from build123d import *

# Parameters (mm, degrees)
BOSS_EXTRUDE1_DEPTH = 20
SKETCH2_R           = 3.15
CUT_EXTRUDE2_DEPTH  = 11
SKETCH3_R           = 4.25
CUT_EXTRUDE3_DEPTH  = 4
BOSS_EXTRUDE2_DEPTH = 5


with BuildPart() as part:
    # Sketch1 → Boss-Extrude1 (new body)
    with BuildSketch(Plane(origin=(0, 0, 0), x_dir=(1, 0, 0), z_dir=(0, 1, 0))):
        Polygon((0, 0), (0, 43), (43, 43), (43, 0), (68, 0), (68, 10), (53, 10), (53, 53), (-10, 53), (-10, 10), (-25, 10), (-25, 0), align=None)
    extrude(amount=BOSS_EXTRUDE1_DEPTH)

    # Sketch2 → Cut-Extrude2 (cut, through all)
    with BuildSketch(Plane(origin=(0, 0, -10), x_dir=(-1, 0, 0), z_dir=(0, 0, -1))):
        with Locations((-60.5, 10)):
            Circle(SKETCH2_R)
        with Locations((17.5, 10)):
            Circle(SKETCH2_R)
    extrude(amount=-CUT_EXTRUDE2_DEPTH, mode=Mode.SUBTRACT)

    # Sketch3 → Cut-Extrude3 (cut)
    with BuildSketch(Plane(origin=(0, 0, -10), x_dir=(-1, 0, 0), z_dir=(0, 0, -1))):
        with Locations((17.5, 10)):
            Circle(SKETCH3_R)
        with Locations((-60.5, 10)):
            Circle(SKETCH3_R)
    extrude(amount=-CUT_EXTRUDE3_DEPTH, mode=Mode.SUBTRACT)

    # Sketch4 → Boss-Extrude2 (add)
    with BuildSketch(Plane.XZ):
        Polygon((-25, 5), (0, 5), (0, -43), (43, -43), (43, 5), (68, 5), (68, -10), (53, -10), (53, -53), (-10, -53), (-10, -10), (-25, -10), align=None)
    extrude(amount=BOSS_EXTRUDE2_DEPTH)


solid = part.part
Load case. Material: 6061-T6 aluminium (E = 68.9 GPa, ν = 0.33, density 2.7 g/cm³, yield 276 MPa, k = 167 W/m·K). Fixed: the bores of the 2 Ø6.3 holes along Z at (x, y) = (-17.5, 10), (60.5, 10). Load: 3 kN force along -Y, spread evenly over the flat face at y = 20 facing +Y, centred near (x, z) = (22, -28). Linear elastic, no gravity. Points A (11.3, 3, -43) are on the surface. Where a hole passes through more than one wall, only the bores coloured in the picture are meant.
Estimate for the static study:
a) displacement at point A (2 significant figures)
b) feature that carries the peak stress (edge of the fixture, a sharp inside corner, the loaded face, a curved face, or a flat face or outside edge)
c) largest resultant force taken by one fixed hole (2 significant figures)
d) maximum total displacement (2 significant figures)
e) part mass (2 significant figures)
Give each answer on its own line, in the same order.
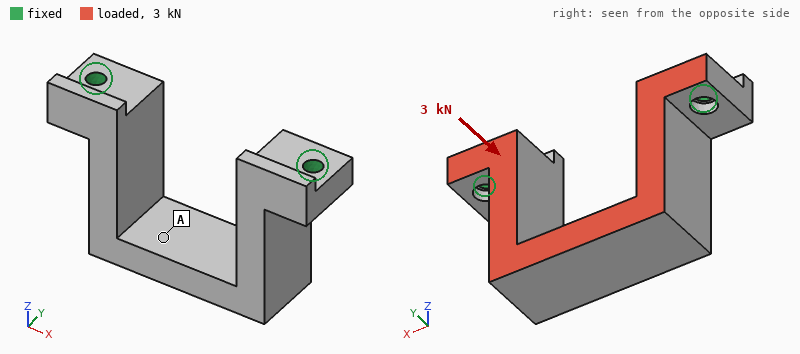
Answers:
0.18 mm
edge of the fixture
1.5 kN
0.23 mm
120 g
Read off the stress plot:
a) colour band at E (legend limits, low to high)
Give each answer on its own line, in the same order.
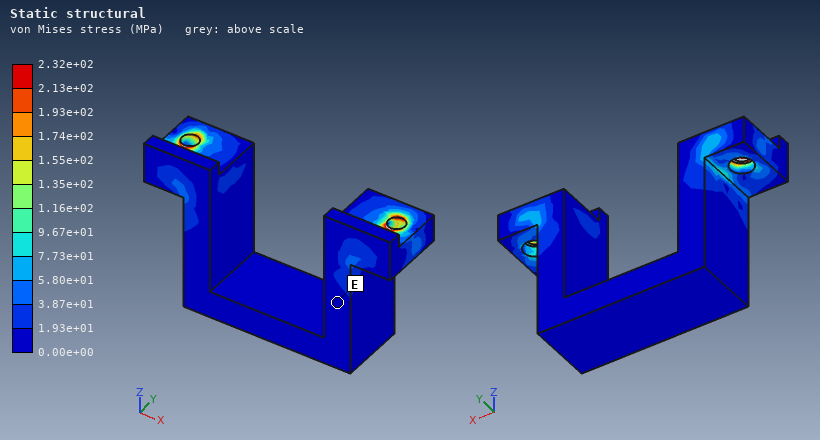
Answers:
0.00e+00 to 1.93e+01 MPa
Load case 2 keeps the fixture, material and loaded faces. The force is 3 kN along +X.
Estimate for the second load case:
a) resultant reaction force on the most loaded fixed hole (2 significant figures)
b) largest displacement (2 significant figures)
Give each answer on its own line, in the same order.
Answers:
1.7 kN
0.10 mm
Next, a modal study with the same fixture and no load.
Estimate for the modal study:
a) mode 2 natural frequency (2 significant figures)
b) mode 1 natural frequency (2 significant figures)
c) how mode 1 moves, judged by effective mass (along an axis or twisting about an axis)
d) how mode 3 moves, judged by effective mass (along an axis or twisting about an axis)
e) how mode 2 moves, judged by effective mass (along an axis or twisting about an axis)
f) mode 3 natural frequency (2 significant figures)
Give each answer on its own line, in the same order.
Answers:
3000 Hz
1900 Hz
along Y
twisting about Z
along X
4100 Hz
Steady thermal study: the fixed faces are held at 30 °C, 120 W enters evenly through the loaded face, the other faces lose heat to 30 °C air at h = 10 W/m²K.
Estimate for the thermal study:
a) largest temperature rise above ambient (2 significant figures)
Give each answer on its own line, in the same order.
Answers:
53 K
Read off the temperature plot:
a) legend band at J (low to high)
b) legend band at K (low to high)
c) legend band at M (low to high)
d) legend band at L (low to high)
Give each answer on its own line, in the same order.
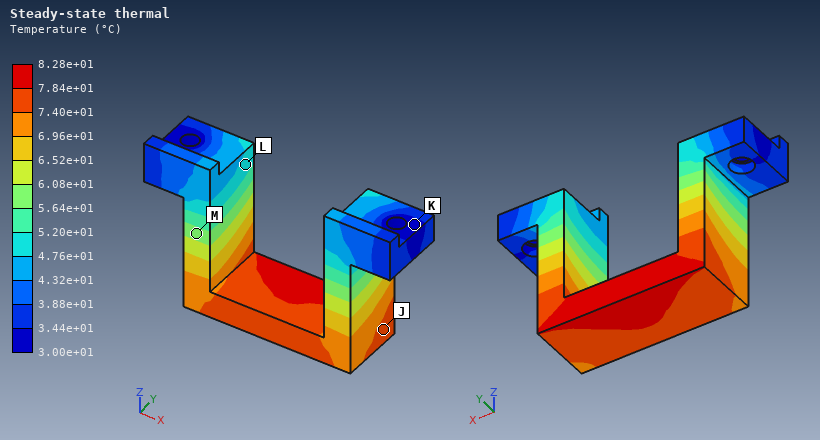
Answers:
7.40e+01 to 7.84e+01 °C
3.00e+01 to 3.44e+01 °C
5.64e+01 to 6.08e+01 °C
4.76e+01 to 5.20e+01 °C
